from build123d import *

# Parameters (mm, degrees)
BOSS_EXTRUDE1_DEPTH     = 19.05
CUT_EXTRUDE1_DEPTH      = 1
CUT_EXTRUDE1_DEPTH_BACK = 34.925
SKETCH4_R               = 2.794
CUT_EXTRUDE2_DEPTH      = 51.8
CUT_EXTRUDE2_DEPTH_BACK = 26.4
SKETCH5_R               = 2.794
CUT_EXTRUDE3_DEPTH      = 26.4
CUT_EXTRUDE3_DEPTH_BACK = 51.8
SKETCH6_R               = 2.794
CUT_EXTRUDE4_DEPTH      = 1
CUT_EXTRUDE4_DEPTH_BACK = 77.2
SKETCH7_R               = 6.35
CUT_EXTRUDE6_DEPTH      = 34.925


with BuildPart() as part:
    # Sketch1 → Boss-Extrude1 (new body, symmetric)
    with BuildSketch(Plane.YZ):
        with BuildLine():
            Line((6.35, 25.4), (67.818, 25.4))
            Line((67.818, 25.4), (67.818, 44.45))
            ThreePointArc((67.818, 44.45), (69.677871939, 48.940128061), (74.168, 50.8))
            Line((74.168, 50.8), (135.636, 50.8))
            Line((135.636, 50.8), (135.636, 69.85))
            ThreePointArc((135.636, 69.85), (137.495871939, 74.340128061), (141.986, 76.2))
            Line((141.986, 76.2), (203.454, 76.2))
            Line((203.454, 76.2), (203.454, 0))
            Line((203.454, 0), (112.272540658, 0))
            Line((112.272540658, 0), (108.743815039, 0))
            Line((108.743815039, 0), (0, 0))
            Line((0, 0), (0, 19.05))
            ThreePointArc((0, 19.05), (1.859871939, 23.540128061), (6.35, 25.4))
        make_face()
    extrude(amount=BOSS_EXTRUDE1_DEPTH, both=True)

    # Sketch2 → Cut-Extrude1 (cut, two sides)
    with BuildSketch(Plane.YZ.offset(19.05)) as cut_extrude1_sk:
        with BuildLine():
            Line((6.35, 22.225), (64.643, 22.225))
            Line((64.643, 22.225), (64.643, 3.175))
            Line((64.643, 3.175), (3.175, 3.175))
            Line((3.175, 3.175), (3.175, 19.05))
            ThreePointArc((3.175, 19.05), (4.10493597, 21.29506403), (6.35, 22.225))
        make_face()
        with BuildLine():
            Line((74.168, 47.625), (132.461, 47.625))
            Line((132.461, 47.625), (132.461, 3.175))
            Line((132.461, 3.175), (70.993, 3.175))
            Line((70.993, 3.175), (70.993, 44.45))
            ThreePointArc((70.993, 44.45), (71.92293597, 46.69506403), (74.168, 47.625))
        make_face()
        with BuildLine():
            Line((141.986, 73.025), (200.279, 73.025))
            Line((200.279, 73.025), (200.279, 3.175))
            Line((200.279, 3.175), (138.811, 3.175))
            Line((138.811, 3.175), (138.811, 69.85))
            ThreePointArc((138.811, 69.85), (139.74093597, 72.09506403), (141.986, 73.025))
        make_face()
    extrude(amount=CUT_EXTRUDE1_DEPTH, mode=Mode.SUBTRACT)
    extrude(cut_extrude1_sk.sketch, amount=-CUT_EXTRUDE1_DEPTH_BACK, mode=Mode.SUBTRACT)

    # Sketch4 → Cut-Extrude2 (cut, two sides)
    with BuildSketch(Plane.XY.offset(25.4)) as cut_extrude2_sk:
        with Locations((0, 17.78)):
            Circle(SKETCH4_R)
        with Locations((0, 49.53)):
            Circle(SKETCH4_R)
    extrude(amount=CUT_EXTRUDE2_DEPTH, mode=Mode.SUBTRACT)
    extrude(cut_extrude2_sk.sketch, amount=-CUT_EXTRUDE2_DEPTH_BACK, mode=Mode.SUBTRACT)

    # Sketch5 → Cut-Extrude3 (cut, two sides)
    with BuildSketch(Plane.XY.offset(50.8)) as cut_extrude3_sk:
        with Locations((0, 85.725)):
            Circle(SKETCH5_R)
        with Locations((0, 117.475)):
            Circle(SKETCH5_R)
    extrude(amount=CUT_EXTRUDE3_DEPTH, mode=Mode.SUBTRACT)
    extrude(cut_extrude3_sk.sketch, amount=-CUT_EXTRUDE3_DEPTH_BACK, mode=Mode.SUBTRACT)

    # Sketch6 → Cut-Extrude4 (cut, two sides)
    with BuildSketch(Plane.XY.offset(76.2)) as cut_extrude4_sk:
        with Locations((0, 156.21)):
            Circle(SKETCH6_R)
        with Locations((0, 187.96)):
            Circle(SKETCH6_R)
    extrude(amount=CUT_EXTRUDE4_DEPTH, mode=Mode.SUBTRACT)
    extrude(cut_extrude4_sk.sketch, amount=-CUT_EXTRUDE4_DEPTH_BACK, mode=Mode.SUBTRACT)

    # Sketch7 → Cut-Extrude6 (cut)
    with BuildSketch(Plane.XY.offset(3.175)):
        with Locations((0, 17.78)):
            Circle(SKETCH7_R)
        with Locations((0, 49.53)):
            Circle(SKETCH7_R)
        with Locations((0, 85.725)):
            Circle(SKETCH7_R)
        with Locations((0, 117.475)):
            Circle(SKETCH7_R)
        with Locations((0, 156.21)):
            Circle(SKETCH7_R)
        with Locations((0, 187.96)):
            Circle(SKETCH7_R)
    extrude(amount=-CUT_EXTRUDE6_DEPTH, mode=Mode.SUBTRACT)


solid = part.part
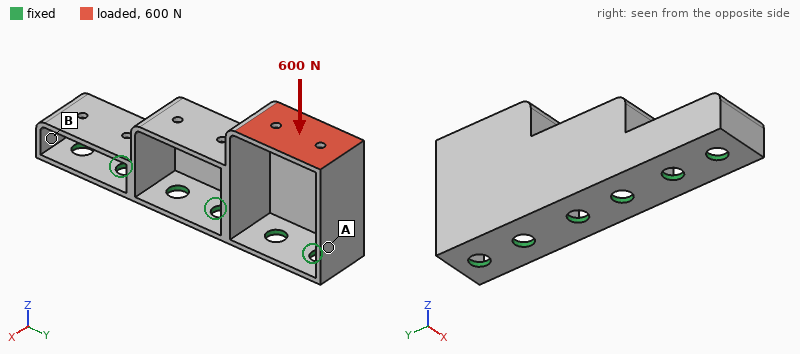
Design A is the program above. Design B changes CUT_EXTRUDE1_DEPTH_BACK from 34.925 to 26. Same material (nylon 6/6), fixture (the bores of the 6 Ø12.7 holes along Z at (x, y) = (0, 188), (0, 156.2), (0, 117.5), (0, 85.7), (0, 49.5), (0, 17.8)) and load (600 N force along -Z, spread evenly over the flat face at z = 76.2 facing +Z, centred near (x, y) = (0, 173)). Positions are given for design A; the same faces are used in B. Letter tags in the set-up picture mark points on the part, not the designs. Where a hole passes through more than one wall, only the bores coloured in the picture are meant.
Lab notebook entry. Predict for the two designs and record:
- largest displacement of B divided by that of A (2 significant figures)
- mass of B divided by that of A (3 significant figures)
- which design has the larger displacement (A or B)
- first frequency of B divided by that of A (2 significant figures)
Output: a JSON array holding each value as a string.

["0.57", "1.70", "A", "0.98"]
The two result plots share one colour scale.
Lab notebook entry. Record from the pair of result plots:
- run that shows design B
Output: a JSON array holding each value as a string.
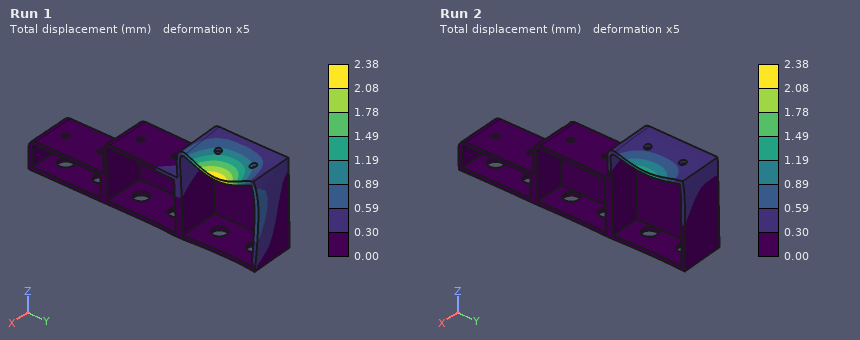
["Run 2"]
